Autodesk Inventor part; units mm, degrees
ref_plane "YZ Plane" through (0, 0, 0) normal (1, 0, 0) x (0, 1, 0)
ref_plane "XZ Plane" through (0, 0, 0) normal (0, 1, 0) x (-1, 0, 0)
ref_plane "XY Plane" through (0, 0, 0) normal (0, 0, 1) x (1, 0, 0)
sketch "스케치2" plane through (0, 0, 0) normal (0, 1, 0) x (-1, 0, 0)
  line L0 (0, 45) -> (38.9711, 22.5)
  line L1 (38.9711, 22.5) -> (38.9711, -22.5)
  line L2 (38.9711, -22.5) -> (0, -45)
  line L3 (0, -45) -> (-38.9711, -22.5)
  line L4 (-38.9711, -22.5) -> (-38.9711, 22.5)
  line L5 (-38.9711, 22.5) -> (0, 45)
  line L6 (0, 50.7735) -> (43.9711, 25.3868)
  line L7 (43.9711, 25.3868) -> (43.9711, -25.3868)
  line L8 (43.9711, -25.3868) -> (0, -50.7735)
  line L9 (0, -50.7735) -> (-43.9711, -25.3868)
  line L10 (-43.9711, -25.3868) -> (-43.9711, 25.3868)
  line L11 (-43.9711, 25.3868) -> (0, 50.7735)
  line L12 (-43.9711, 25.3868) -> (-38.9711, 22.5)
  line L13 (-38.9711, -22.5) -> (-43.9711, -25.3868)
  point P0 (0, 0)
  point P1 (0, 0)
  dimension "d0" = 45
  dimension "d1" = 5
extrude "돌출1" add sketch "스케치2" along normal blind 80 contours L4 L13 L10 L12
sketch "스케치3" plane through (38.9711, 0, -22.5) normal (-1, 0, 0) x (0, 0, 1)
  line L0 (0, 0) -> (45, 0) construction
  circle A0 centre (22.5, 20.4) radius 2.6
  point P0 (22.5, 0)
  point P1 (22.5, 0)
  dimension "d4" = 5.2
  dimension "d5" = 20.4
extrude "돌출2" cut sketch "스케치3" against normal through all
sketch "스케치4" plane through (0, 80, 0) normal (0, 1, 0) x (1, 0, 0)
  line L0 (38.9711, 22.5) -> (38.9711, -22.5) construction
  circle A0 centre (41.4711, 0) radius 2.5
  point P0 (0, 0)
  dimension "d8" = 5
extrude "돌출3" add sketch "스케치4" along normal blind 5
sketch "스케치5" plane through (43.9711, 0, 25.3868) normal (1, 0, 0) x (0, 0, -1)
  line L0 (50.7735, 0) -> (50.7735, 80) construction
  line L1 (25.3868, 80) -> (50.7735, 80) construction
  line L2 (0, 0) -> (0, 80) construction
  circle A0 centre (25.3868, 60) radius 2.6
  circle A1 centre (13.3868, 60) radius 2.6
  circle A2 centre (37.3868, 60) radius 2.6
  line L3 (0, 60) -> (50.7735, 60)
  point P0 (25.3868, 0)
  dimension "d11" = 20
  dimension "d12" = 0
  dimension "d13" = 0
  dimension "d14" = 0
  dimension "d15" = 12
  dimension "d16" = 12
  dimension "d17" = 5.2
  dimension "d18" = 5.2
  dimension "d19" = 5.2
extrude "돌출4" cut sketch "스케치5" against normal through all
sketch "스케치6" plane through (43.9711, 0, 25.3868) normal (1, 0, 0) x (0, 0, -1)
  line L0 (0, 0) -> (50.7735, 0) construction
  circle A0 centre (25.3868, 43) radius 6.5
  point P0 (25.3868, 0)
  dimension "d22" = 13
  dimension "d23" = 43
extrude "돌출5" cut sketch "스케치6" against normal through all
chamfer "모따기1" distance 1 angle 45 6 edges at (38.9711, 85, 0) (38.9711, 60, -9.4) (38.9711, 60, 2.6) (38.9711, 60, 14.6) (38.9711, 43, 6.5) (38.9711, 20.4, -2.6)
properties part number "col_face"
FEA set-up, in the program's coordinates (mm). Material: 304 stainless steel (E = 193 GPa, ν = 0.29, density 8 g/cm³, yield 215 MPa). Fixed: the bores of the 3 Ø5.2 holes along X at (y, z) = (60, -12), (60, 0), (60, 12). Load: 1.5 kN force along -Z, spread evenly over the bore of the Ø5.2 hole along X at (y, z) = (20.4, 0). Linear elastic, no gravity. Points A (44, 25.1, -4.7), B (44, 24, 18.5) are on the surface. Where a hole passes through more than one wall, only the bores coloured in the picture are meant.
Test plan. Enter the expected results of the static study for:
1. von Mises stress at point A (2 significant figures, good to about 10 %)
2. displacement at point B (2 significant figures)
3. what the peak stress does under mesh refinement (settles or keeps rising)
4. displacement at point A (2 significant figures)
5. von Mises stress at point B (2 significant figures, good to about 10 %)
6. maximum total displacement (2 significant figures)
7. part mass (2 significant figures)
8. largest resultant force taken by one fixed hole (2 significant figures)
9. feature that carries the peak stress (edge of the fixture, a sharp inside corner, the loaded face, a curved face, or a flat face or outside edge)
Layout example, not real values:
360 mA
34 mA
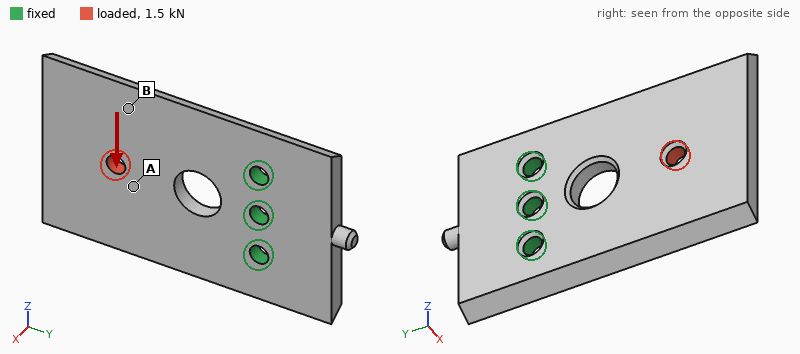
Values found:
22 MPa
13 µm
keeps rising
11 µm
6.5 MPa
19 µm
140 g
2.1 kN
edge of the fixture
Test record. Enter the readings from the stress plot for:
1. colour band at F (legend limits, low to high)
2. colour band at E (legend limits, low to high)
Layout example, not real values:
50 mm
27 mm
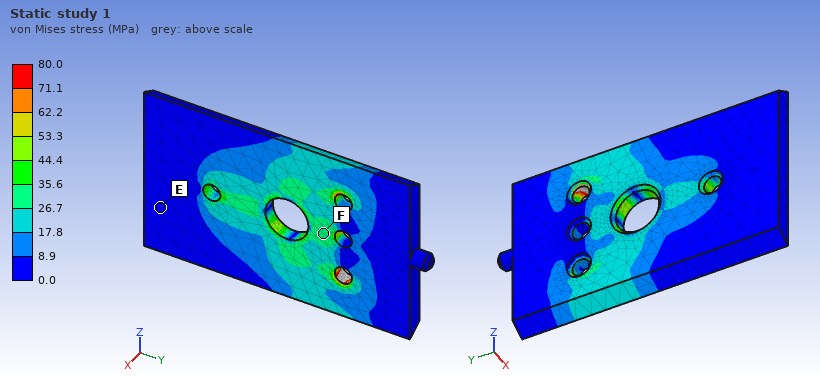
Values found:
26.7 to 35.6 MPa
0.0 to 8.9 MPa
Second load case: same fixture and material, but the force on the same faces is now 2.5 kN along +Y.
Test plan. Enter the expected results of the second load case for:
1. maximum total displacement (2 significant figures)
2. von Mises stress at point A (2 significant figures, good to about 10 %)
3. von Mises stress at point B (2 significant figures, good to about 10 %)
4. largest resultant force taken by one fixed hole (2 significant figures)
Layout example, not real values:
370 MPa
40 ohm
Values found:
21 µm
27 MPa
11 MPa
1.1 kN
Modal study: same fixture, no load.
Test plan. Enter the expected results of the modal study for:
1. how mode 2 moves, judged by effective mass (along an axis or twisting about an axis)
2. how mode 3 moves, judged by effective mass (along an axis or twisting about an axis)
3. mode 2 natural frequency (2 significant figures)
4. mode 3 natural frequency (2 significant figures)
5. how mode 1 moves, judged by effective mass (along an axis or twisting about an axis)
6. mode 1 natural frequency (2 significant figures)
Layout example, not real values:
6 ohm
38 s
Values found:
twisting about Y
along Z
2900 Hz
6000 Hz
along X
1000 Hz
